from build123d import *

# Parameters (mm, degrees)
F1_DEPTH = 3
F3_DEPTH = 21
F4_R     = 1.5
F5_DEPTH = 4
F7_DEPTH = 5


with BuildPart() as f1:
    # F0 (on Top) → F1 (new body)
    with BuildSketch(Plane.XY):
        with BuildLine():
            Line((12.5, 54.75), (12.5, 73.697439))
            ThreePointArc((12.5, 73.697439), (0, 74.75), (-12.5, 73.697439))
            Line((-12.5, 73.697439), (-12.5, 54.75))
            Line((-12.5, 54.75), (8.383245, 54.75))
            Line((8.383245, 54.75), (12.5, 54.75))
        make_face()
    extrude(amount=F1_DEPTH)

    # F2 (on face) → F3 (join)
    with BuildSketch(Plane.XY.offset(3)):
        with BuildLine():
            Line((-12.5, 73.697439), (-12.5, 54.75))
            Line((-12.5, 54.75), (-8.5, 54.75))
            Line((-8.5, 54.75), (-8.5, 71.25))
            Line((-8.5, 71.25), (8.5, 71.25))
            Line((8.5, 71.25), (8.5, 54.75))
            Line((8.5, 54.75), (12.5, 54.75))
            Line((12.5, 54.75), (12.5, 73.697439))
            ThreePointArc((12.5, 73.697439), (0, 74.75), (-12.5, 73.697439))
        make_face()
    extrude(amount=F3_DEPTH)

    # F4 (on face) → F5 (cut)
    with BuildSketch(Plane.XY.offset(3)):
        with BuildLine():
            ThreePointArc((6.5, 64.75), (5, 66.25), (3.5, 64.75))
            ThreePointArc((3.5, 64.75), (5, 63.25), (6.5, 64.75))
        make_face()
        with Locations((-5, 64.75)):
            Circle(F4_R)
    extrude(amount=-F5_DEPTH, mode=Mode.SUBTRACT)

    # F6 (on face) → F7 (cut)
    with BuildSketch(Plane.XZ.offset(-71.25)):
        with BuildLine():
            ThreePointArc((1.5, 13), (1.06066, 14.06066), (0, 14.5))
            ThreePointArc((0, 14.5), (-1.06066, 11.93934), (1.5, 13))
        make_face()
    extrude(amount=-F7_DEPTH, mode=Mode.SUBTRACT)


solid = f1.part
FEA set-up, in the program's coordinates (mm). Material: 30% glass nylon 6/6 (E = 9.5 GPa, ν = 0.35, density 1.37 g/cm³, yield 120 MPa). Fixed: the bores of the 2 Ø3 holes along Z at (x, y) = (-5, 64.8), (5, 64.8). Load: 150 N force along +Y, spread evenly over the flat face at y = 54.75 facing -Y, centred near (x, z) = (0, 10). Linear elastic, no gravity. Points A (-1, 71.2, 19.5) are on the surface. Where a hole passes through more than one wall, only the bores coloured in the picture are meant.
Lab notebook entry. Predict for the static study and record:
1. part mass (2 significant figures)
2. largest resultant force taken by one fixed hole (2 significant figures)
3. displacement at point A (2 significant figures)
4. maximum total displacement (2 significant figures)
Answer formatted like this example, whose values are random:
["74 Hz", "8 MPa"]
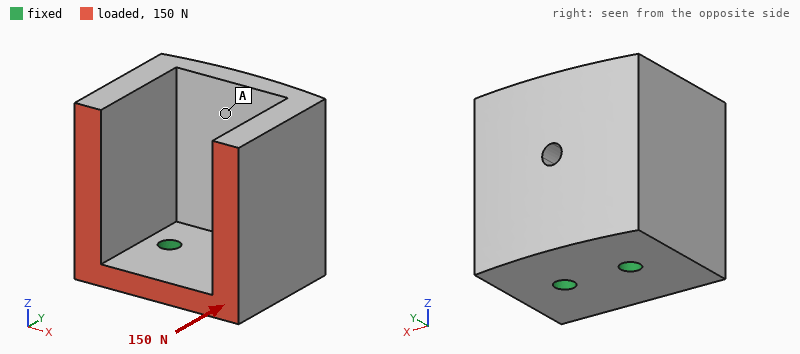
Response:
["8.0 g", "75 N", "0.081 mm", "0.11 mm"]
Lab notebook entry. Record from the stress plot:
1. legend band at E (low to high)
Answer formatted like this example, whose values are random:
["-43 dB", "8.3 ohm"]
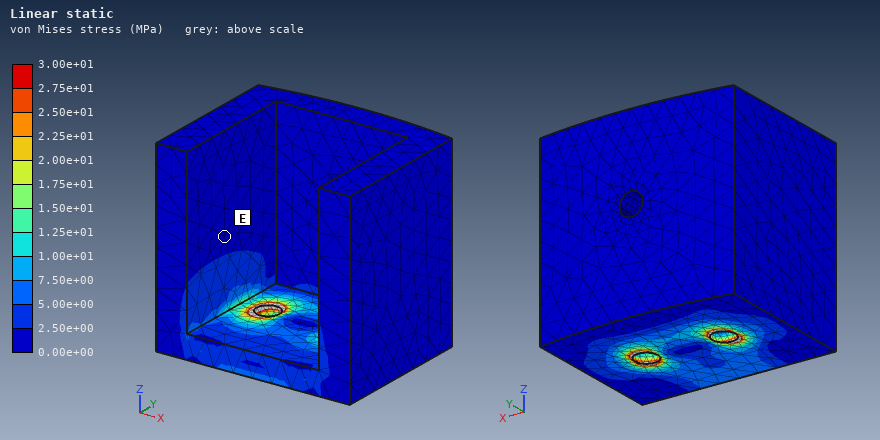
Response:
["0.00e+00 to 2.50e+00 MPa"]
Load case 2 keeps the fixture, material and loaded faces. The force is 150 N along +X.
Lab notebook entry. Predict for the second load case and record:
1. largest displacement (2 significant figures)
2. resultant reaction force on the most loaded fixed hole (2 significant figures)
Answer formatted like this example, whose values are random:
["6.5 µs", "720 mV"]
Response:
["0.16 mm", "150 N"]
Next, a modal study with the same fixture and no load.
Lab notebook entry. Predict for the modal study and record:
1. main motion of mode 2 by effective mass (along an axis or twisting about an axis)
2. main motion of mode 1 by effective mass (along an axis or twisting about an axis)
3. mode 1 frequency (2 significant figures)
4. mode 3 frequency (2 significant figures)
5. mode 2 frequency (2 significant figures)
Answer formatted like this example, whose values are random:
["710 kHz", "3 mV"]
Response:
["along X", "along Y", "2300 Hz", "5100 Hz", "2700 Hz"]
